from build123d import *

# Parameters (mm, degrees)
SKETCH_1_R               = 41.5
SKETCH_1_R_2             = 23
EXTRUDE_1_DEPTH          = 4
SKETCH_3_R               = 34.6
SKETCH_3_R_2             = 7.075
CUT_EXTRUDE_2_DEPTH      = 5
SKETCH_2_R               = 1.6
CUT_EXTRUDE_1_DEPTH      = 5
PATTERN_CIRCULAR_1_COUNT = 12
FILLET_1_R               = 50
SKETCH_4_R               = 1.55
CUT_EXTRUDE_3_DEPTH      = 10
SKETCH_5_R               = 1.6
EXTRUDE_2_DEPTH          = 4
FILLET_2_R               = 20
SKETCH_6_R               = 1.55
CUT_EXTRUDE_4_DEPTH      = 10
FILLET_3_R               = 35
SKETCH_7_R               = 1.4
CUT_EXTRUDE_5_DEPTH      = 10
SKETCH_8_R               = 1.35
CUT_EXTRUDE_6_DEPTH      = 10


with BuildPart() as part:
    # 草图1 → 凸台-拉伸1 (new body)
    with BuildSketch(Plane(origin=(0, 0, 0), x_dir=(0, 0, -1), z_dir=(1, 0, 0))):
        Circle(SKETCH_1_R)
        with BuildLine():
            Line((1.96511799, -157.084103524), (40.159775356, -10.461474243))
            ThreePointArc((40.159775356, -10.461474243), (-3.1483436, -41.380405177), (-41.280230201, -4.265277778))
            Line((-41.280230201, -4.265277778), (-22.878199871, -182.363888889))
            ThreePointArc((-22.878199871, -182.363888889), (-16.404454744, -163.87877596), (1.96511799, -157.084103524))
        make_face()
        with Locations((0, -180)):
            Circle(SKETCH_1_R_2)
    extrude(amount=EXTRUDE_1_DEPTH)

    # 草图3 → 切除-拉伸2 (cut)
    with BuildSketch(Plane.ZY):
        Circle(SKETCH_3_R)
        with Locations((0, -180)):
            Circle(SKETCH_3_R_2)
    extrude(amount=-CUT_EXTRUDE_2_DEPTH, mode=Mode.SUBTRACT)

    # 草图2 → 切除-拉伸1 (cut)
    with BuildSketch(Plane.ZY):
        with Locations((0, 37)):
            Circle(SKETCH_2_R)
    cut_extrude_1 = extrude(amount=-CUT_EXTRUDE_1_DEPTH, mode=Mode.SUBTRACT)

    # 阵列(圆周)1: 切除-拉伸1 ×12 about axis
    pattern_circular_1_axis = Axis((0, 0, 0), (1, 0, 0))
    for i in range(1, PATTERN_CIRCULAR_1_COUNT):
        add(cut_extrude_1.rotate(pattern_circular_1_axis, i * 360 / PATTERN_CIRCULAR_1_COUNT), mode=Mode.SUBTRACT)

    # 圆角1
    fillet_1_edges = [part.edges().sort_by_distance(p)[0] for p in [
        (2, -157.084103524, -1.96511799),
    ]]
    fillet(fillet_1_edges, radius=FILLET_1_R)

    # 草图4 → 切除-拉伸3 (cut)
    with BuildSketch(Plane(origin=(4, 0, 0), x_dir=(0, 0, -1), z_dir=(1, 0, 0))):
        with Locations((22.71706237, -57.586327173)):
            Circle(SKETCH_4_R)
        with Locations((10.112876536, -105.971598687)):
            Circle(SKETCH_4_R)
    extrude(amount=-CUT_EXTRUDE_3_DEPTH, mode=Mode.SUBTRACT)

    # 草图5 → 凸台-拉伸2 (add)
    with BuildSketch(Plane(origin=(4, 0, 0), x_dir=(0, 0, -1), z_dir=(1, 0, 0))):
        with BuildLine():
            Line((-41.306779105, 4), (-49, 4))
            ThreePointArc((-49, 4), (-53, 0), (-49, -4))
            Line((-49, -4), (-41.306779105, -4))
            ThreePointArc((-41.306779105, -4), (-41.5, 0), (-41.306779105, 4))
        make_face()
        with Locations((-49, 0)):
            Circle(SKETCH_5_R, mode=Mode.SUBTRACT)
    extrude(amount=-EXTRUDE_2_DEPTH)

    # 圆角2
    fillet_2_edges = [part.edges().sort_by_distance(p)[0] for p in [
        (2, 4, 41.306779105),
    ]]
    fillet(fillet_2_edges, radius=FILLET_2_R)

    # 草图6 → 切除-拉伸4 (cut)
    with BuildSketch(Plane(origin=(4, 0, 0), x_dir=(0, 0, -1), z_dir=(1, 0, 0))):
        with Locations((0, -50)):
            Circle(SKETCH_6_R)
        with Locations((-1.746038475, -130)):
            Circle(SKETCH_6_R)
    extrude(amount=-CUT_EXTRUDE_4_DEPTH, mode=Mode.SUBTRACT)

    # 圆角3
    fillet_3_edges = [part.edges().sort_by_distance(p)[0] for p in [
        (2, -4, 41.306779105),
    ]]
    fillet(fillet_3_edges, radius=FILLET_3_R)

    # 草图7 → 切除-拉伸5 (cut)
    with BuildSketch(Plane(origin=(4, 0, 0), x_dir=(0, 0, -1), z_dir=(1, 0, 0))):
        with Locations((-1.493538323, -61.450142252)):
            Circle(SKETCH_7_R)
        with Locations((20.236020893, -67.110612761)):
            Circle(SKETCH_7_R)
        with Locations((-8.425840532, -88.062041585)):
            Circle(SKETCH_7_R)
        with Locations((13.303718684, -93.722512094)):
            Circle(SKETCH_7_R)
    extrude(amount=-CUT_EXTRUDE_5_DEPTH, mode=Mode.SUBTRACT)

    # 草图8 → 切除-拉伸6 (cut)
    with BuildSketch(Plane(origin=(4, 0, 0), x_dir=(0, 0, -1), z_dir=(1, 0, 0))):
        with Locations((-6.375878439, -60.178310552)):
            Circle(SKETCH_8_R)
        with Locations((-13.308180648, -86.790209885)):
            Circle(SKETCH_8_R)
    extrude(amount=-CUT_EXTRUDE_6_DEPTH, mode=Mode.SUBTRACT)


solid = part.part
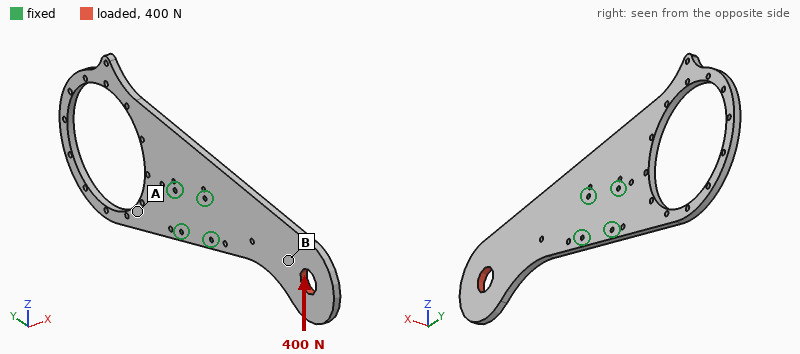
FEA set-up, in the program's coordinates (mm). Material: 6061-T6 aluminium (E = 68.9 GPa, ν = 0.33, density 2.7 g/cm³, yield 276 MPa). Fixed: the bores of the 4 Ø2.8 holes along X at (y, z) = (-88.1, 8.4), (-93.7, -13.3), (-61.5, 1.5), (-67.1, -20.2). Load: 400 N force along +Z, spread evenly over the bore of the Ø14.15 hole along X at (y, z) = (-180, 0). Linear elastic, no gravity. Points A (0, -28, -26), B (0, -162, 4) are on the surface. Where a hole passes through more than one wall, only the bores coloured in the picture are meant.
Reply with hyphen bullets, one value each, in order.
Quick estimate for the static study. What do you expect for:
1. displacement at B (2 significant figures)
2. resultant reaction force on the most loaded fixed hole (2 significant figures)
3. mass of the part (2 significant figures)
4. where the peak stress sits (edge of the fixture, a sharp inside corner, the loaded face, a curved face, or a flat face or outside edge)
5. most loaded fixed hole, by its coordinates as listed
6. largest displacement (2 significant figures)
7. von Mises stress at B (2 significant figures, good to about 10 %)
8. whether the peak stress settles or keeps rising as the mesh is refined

- 0.055 mm
- 1.0 kN
- 100 g
- edge of the fixture
- (-93.7, -13.3)
- 0.11 mm
- 8.2 MPa
- keeps rising
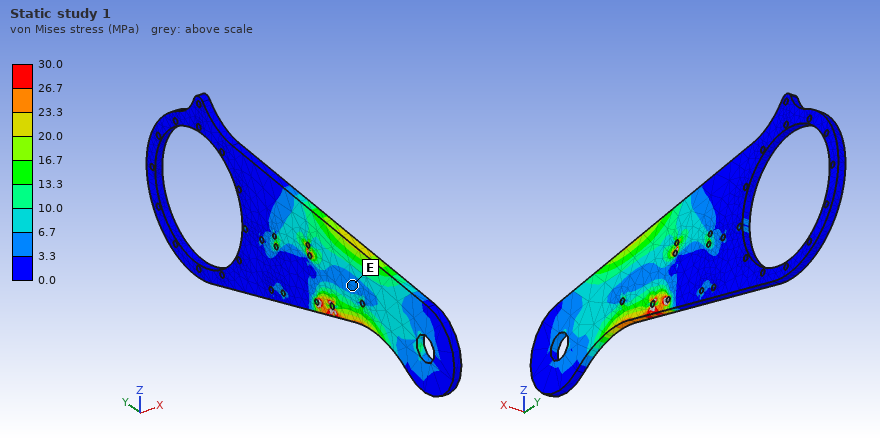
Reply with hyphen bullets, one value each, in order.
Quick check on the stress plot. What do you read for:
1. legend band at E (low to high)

- 3.3 to 6.7 MPa
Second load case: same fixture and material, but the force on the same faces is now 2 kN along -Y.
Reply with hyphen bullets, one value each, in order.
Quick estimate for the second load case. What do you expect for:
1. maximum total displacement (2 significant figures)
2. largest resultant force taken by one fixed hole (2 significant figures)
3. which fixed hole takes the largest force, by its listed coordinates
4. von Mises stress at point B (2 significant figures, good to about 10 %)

- 65 µm
- 940 N
- (-88.1, 8.4)
- 16 MPa
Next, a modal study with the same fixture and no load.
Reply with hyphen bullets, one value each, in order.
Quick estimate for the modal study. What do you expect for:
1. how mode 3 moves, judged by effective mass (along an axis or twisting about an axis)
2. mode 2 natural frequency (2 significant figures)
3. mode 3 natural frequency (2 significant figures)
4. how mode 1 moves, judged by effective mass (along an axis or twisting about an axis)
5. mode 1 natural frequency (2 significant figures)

- twisting about Y
- 360 Hz
- 730 Hz
- along X
- 280 Hz
